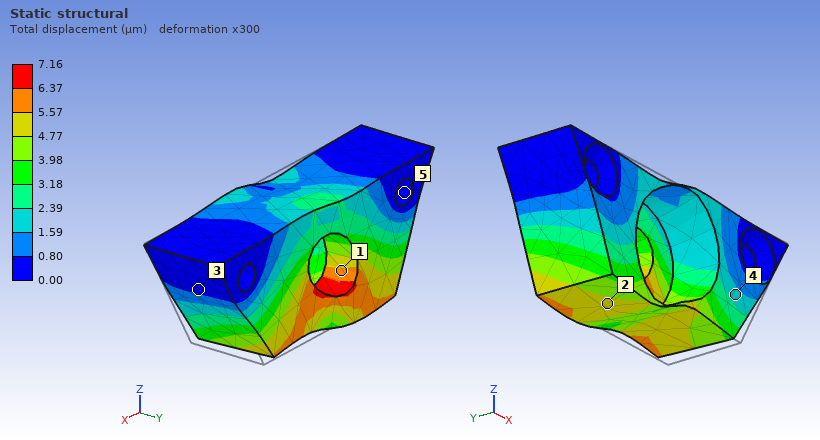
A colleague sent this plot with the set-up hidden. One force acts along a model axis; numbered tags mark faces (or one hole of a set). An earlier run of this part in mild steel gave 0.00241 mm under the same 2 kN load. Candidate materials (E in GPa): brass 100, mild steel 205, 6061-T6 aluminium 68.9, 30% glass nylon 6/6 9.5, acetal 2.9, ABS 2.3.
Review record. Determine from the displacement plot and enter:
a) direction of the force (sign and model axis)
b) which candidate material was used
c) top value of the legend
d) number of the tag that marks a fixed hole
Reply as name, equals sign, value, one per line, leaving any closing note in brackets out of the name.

direction of the force = -X
which candidate material was used = 6061-T6 aluminium
top value of the legend = 7.16 µm
number of the tag that marks a fixed hole = 5
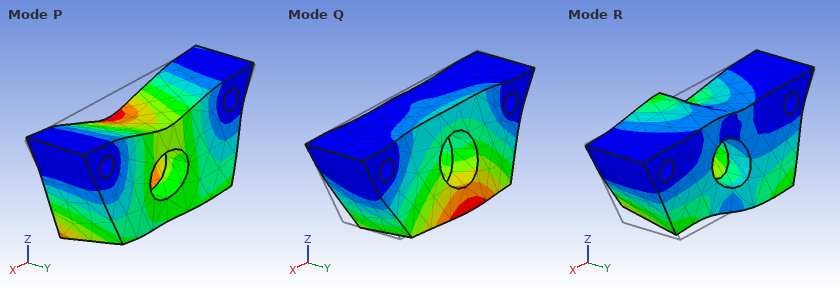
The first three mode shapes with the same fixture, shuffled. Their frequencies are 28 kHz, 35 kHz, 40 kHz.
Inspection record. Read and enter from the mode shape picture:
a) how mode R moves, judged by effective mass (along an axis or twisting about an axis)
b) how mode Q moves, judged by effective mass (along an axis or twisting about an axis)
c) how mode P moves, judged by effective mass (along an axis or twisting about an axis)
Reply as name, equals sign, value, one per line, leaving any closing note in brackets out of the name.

how mode R moves, judged by effective mass = along X
how mode Q moves, judged by effective mass = along Y
how mode P moves, judged by effective mass = along Z
